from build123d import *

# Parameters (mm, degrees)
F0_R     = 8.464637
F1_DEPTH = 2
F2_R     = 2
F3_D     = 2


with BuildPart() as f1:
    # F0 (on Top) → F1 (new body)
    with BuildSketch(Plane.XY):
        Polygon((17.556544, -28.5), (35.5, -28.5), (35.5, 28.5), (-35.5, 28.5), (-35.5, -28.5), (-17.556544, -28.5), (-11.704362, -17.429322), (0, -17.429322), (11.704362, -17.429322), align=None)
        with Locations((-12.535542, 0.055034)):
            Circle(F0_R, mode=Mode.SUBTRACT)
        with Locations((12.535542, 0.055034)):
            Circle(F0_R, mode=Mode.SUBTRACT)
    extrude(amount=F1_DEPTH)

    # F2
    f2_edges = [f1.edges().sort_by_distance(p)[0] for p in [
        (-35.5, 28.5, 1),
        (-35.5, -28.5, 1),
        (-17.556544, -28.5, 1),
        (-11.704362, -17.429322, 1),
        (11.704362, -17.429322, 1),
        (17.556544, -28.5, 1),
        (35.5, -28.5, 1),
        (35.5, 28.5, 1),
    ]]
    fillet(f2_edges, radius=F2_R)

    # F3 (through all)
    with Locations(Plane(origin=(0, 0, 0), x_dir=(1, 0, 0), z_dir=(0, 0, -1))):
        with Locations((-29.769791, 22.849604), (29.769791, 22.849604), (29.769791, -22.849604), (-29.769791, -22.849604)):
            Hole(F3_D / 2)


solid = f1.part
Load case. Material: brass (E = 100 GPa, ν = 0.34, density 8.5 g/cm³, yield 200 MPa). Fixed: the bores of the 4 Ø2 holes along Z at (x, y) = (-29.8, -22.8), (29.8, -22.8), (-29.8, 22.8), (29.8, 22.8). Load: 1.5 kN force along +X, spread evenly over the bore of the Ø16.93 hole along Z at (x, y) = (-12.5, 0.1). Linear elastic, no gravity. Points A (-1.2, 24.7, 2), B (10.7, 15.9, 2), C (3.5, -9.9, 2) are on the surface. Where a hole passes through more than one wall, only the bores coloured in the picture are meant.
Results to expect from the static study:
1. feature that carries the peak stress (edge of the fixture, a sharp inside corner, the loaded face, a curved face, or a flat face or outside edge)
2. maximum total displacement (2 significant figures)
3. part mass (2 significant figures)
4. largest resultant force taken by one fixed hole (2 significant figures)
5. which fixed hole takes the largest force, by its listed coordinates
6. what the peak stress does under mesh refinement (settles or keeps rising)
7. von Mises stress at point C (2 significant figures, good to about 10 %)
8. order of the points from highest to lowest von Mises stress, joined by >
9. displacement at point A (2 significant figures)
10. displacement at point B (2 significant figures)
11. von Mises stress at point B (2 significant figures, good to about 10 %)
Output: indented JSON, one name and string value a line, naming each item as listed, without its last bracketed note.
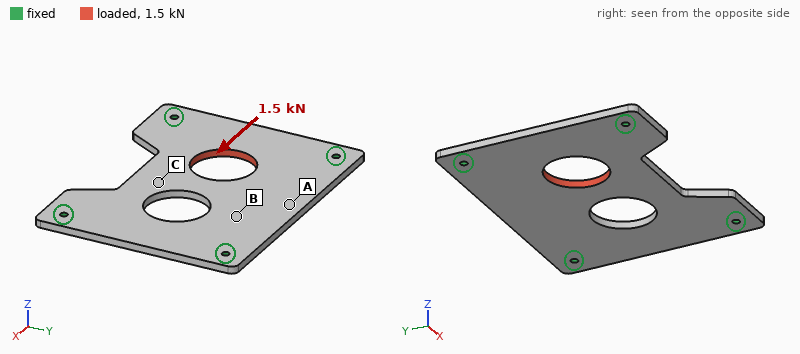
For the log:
{
  "feature that carries the peak stress": "edge of the fixture",
  "maximum total displacement": "9.4 µm",
  "part mass": "55 g",
  "largest resultant force taken by one fixed hole": "510 N",
  "which fixed hole takes the largest force, by its listed coordinates": "(-29.8, 22.8)",
  "what the peak stress does under mesh refinement": "keeps rising",
  "von Mises stress at point C": "14 MPa",
  "order of the points from highest to lowest von Mises stress, joined by >": "C > B > A",
  "displacement at point A": "3.1 µm",
  "displacement at point B": "3.0 µm",
  "von Mises stress at point B": "11 MPa"
}
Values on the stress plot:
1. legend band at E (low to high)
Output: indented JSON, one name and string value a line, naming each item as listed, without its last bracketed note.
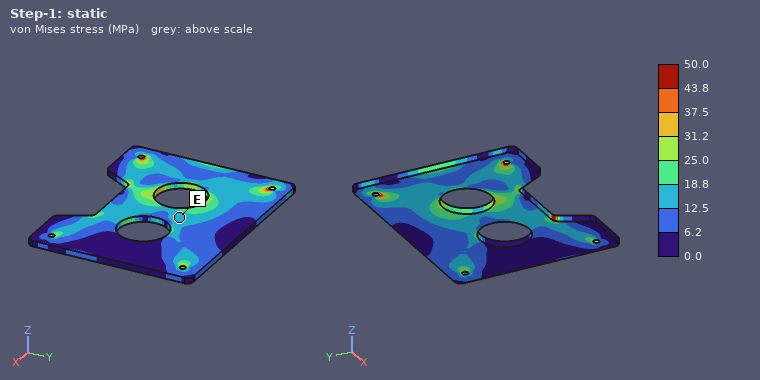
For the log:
{
  "legend band at E": "12.5 to 18.8 MPa"
}
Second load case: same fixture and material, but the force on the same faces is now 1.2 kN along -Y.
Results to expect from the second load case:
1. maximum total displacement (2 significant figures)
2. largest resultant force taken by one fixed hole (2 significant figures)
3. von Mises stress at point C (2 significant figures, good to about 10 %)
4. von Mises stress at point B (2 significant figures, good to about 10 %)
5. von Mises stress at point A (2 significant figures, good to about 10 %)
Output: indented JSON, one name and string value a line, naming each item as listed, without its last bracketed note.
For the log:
{
  "maximum total displacement": "8.4 µm",
  "largest resultant force taken by one fixed hole": "490 N",
  "von Mises stress at point C": "8.6 MPa",
  "von Mises stress at point B": "11 MPa",
  "von Mises stress at point A": "7.8 MPa"
}
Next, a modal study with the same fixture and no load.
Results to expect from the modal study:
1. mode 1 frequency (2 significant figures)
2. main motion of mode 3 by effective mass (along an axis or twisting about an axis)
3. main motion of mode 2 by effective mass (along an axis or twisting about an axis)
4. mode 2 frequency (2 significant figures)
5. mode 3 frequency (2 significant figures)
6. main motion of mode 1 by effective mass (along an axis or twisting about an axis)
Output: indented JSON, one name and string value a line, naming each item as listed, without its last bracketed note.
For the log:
{
  "mode 1 frequency": "1600 Hz",
  "main motion of mode 3 by effective mass": "twisting about Y",
  "main motion of mode 2 by effective mass": "twisting about X",
  "mode 2 frequency": "2400 Hz",
  "mode 3 frequency": "3200 Hz",
  "main motion of mode 1 by effective mass": "along Z"
}
